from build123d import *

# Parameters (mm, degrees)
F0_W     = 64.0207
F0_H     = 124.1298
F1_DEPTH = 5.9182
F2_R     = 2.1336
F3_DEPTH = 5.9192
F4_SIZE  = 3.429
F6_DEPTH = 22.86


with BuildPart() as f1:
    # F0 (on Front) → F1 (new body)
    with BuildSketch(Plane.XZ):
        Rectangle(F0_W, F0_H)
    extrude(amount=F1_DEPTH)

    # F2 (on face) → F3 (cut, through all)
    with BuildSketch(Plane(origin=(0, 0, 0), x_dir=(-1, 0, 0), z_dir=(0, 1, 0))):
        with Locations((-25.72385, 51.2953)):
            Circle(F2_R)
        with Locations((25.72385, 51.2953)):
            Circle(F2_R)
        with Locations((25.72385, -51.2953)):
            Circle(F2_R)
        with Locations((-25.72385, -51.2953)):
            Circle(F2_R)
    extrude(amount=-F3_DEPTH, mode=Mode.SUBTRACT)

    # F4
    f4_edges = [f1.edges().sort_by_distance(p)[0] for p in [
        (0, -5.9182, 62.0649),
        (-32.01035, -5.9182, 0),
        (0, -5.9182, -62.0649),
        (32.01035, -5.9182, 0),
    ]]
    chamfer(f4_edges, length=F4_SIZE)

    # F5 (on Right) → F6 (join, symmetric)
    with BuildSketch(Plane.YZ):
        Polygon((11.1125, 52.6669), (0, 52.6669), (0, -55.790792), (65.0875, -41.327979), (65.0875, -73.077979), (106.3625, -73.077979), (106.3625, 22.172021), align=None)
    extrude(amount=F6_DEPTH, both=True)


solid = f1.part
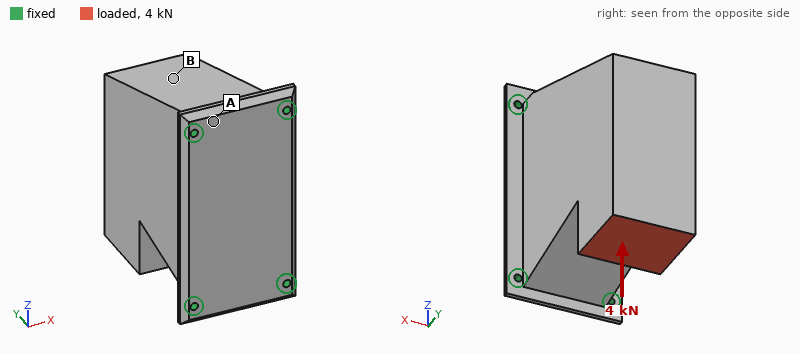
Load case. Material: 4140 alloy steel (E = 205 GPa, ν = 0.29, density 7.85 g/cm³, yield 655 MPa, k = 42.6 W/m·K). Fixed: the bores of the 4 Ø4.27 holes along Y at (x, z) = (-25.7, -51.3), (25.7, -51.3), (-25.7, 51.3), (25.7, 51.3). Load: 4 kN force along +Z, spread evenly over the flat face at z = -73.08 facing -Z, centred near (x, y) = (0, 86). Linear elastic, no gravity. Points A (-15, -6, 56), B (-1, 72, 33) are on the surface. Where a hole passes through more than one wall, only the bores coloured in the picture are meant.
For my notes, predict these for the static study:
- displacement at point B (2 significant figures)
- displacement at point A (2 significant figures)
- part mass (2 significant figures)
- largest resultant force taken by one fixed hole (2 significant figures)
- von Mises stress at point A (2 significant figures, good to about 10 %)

6.9 µm
2.7 µm
4.1 kg
2.2 kN
11 MPa
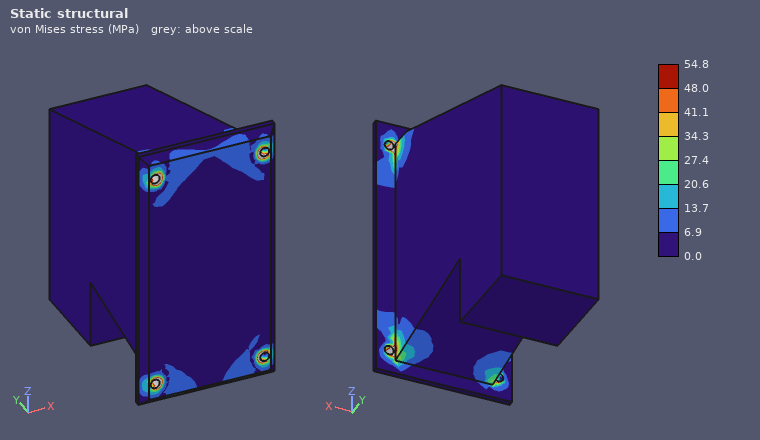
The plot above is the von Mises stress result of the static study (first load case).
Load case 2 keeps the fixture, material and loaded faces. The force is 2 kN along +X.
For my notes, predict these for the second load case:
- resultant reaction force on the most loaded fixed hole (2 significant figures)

2.6 kN
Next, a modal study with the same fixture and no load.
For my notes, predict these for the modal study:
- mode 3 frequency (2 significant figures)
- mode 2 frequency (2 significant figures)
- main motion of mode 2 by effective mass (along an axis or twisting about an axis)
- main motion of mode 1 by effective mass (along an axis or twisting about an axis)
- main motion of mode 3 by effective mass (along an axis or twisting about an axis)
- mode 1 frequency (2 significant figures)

3500 Hz
2400 Hz
along Z
along X
along Y
1200 Hz
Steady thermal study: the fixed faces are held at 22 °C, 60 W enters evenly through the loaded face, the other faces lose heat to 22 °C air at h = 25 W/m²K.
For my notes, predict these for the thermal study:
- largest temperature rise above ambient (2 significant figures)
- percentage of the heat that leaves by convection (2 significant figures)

68 K
51 %
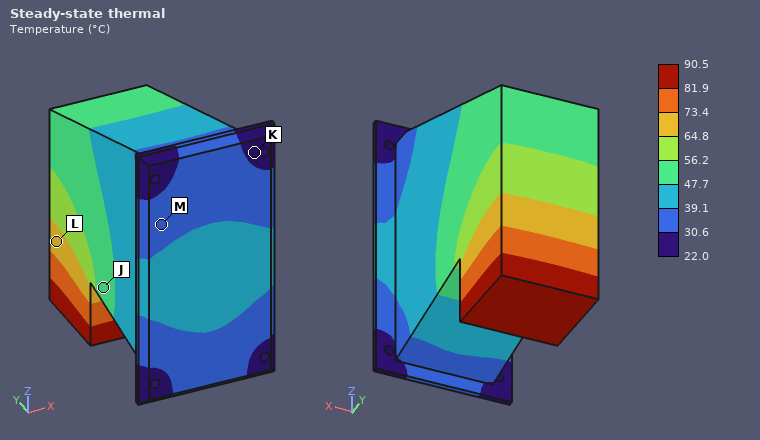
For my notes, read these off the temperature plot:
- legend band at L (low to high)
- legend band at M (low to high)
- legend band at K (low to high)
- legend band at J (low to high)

64.8 to 73.4 °C
30.6 to 39.1 °C
22.0 to 30.6 °C
47.7 to 56.2 °C
